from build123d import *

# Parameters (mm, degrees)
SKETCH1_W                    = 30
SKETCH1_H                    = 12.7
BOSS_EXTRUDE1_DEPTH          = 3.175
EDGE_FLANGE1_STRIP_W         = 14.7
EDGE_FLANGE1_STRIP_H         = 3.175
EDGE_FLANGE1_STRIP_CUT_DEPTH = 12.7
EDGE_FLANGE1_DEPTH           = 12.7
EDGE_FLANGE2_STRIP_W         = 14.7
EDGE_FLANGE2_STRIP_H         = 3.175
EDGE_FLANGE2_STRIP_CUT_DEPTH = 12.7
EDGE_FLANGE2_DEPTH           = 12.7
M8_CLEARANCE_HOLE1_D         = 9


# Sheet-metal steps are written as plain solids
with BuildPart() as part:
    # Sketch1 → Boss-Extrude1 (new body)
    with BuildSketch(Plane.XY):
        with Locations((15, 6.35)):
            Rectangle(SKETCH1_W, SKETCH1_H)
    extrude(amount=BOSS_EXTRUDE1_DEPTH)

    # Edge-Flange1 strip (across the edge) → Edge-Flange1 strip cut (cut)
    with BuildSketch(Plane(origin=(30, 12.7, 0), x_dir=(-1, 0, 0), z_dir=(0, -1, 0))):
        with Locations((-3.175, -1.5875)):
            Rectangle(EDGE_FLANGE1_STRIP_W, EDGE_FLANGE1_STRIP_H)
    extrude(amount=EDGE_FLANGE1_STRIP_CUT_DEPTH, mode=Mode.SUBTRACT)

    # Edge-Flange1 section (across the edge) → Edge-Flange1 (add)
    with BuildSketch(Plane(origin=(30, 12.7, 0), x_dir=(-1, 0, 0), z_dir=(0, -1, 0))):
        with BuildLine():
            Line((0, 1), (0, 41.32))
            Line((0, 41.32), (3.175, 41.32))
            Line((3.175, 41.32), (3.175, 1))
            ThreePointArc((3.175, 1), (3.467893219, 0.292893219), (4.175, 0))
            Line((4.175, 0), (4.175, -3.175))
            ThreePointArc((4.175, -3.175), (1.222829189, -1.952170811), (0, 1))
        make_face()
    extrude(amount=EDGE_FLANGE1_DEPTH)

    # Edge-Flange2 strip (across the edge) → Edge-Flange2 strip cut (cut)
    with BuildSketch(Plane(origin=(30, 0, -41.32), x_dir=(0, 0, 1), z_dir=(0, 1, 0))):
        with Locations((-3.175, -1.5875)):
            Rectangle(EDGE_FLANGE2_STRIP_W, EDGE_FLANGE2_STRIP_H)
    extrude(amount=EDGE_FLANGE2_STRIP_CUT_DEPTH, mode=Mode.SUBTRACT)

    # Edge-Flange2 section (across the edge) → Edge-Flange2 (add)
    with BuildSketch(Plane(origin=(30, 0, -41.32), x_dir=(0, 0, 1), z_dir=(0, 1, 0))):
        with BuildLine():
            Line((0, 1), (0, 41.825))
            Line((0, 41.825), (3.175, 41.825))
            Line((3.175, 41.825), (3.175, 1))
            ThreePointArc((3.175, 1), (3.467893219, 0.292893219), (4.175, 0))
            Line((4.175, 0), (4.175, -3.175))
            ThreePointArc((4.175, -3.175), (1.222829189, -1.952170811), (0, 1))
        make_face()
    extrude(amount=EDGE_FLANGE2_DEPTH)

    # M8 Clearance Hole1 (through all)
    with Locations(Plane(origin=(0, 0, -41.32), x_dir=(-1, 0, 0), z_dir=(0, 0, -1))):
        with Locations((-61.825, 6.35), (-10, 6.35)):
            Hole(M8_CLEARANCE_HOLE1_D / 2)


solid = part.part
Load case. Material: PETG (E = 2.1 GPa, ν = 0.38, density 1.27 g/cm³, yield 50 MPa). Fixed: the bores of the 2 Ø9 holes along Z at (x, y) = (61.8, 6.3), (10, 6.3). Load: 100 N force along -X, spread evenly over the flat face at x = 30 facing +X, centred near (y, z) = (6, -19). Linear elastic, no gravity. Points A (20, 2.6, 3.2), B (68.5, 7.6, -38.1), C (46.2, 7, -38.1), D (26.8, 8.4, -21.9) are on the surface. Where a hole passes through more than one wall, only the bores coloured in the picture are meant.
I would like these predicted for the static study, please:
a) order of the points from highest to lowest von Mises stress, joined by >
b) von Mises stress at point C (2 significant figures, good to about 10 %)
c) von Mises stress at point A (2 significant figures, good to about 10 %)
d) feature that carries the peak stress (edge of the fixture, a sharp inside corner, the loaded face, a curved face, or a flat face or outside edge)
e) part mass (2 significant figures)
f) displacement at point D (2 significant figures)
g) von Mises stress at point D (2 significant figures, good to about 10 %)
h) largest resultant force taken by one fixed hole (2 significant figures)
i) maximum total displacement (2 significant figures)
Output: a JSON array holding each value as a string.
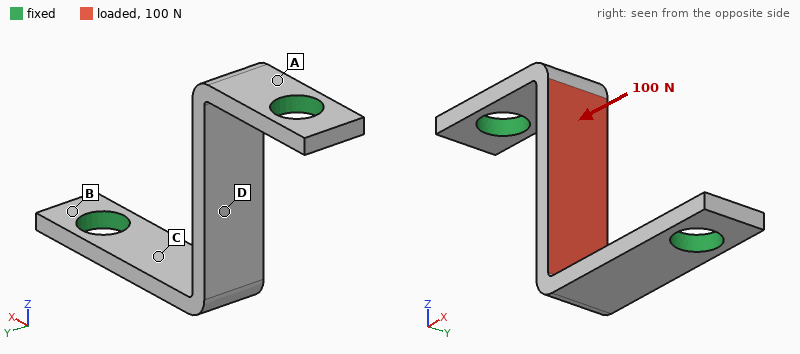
["D > A > C > B", "5.4 MPa", "11 MPa", "a curved face", "5.2 g", "0.87 mm", "16 MPa", "52 N", "0.91 mm"]
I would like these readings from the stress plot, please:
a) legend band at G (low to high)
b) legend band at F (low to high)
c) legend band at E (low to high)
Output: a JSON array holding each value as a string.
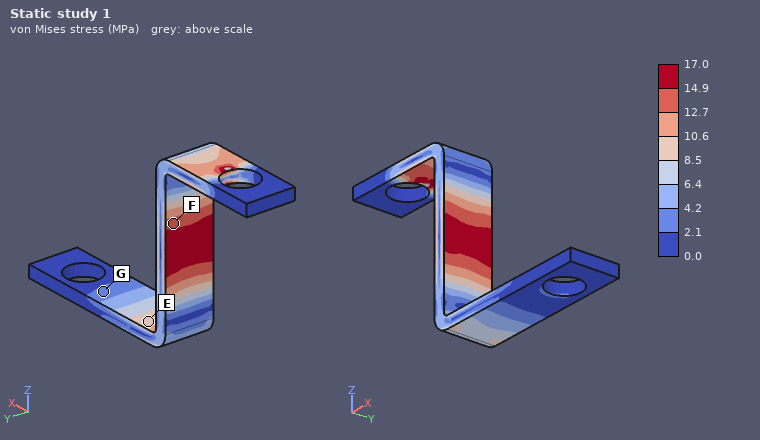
["2.1 to 4.2 MPa", "12.7 to 14.9 MPa", "8.5 to 10.6 MPa"]
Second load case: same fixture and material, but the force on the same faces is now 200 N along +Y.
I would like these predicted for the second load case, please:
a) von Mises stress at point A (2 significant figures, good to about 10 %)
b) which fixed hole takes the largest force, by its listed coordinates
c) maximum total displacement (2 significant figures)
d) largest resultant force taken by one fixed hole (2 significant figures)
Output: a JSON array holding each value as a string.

["8.0 MPa", "(10, 6.3)", "0.93 mm", "110 N"]
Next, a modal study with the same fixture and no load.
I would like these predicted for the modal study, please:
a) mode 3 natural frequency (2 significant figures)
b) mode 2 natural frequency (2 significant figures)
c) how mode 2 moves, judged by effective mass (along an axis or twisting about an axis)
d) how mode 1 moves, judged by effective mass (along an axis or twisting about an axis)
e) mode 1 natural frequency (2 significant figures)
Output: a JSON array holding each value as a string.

["2000 Hz", "1500 Hz", "along Y", "along Z", "970 Hz"]
